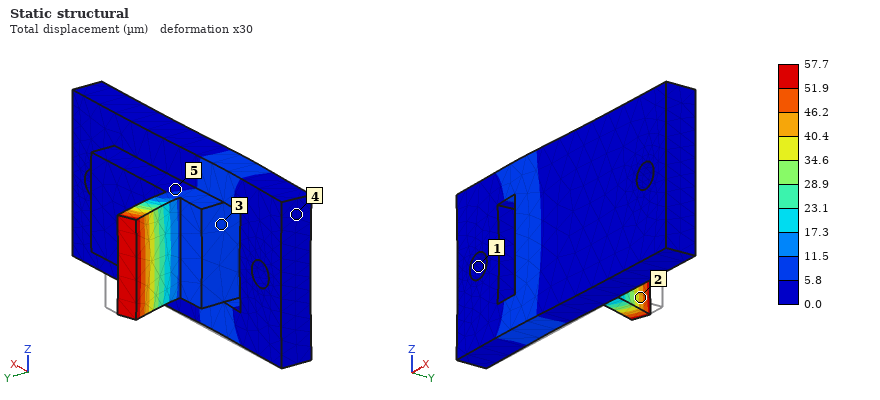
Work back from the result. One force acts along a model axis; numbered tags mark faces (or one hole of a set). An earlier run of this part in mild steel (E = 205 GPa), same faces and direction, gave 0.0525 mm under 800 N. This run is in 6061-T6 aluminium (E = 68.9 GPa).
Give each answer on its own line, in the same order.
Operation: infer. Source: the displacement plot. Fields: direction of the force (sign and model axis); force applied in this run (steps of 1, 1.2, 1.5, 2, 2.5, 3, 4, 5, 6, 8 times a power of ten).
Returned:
-X
300 N
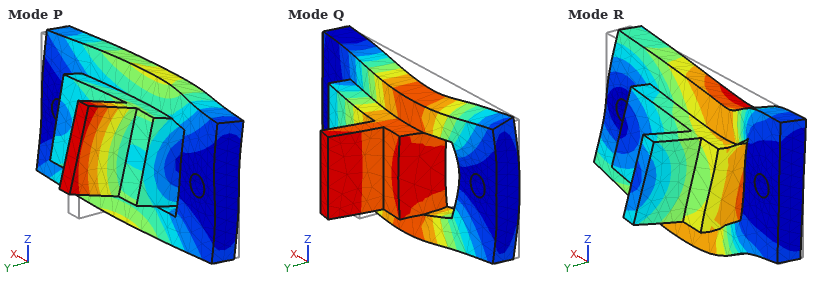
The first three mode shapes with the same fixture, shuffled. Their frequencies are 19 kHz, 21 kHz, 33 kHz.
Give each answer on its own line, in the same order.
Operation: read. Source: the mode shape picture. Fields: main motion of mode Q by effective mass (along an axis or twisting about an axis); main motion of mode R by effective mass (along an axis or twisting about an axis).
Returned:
along Y
along Z
